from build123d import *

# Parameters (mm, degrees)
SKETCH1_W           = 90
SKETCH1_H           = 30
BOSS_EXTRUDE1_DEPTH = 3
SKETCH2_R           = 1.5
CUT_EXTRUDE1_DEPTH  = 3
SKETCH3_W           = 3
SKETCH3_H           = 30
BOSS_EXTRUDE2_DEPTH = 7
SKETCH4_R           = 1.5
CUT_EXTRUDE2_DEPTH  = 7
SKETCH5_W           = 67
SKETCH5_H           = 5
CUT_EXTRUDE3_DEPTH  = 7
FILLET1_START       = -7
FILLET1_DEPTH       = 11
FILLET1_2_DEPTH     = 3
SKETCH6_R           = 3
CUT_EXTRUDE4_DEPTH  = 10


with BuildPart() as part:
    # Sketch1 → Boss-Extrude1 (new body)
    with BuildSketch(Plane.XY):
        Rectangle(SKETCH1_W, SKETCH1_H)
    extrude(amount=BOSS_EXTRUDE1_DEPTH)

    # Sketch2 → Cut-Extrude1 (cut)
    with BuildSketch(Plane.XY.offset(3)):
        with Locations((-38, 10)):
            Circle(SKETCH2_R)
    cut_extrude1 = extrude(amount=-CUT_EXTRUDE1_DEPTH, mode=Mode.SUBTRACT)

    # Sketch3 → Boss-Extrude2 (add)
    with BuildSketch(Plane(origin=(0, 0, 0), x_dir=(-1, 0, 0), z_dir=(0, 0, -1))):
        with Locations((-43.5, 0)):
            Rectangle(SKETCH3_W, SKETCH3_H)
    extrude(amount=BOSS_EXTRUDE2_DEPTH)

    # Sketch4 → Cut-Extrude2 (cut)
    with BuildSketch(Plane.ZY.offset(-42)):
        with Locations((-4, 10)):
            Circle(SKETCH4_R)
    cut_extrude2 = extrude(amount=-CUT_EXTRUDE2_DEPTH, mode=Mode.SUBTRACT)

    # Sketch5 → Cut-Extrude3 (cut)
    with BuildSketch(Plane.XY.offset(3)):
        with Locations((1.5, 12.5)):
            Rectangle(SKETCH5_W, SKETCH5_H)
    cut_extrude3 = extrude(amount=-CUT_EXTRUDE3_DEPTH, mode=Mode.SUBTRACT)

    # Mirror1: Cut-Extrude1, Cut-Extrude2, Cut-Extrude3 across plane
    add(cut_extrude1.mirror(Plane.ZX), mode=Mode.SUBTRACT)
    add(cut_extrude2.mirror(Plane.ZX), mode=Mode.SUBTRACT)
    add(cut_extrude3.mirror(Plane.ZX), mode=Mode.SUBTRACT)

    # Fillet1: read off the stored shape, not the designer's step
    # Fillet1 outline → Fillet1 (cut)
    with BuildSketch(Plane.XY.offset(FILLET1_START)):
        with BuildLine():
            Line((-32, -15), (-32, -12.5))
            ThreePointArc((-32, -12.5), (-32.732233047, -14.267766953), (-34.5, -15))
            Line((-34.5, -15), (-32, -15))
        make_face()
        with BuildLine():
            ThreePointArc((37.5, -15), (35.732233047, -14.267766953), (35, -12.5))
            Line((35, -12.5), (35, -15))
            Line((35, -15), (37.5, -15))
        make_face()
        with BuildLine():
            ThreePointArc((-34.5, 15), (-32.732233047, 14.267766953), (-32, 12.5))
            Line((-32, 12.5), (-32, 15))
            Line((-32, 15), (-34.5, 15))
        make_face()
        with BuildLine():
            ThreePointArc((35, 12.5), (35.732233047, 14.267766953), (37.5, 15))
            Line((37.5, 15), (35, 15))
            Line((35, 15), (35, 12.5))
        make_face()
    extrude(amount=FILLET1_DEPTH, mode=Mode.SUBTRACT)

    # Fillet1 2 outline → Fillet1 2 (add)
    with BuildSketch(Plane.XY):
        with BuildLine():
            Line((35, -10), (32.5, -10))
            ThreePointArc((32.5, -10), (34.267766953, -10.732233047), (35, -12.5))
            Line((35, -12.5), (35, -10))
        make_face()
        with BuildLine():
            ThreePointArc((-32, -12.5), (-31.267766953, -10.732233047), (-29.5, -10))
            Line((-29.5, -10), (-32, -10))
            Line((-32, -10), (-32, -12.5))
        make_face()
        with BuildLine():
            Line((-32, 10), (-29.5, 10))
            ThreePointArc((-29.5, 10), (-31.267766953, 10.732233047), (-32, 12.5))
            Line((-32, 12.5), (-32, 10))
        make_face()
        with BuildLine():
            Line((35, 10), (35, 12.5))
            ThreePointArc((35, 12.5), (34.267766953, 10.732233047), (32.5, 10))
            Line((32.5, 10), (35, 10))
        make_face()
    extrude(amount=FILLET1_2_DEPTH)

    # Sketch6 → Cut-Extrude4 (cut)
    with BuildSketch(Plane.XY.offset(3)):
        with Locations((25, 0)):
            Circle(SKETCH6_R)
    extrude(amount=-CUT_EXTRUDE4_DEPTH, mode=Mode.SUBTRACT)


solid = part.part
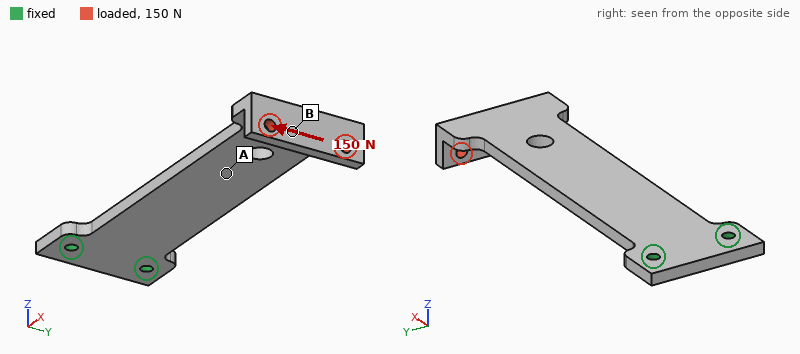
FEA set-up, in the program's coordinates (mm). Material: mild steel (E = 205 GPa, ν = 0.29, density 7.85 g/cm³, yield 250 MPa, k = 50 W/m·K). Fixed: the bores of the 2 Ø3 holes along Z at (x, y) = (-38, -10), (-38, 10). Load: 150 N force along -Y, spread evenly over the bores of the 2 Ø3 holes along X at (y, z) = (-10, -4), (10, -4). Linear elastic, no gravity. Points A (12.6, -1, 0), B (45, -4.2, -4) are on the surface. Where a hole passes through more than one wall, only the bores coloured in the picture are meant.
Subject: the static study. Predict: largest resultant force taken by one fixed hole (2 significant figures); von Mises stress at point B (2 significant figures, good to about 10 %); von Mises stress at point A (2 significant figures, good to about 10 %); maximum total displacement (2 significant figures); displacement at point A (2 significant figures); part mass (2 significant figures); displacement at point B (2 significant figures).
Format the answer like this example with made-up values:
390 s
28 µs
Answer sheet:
610 N
5.5 MPa
34 MPa
0.13 mm
0.032 mm
51 g
0.092 mm
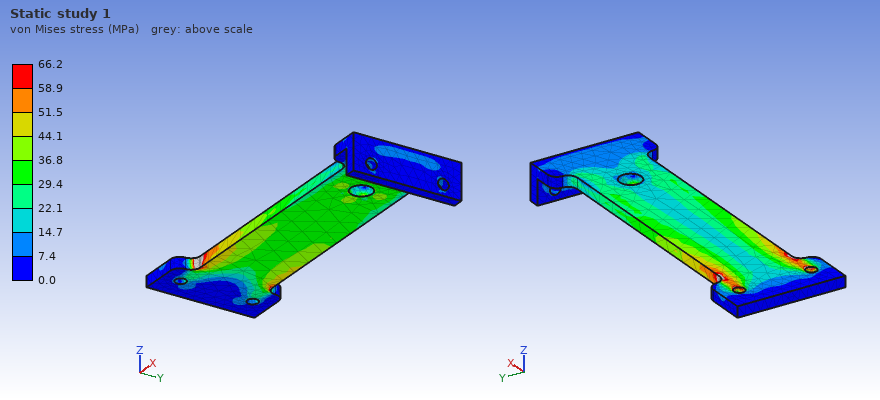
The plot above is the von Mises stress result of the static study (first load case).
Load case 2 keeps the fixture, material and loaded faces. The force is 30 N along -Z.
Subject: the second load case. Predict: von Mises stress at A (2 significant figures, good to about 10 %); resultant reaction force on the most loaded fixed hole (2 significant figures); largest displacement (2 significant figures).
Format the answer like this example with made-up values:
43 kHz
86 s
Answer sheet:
31 MPa
15 N
0.60 mm
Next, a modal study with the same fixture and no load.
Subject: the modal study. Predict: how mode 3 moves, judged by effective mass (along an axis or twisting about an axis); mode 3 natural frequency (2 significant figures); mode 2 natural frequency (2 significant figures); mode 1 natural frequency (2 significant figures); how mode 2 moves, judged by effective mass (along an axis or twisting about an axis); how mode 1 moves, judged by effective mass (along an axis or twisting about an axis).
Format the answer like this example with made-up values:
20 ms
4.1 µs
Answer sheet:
along Z
1900 Hz
1800 Hz
290 Hz
along Y
along Z
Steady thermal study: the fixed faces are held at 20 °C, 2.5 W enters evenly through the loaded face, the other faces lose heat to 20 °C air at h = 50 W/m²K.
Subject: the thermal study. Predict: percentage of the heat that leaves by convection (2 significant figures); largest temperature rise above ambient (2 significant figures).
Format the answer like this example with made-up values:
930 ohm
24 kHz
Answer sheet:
87 %
24 K
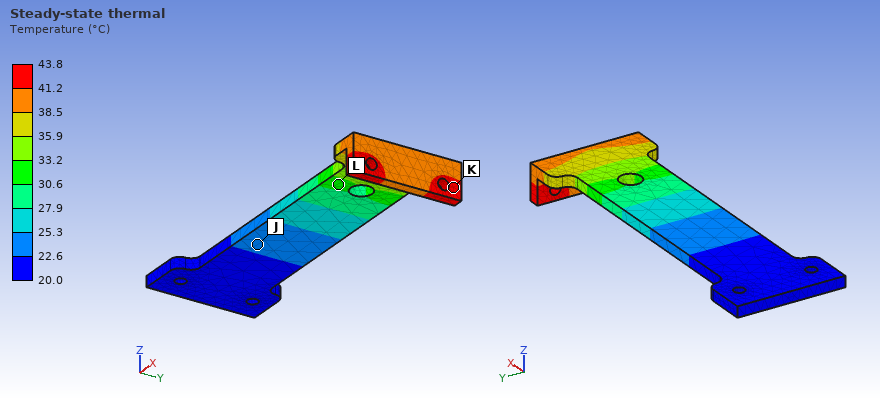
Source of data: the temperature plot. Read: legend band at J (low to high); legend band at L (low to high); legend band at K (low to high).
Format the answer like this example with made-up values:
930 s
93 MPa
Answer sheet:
22.6 to 25.3 °C
30.6 to 33.2 °C
41.2 to 43.8 °C
